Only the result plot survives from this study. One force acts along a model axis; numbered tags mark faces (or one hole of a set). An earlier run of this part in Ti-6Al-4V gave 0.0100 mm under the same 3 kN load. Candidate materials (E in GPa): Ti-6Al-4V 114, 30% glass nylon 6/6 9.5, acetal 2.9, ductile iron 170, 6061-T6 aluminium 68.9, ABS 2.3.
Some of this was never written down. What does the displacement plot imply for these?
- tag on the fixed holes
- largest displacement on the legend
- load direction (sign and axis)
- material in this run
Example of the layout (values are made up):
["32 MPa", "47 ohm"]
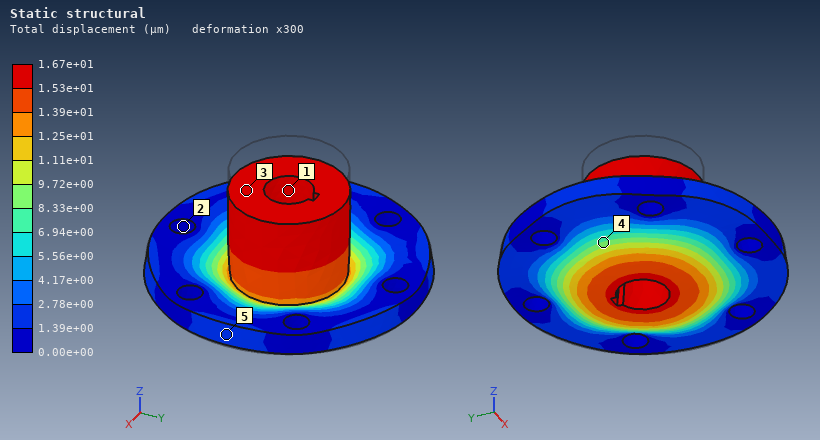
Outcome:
["2", "1.67e+01 µm", "-Z", "6061-T6 aluminium"]
